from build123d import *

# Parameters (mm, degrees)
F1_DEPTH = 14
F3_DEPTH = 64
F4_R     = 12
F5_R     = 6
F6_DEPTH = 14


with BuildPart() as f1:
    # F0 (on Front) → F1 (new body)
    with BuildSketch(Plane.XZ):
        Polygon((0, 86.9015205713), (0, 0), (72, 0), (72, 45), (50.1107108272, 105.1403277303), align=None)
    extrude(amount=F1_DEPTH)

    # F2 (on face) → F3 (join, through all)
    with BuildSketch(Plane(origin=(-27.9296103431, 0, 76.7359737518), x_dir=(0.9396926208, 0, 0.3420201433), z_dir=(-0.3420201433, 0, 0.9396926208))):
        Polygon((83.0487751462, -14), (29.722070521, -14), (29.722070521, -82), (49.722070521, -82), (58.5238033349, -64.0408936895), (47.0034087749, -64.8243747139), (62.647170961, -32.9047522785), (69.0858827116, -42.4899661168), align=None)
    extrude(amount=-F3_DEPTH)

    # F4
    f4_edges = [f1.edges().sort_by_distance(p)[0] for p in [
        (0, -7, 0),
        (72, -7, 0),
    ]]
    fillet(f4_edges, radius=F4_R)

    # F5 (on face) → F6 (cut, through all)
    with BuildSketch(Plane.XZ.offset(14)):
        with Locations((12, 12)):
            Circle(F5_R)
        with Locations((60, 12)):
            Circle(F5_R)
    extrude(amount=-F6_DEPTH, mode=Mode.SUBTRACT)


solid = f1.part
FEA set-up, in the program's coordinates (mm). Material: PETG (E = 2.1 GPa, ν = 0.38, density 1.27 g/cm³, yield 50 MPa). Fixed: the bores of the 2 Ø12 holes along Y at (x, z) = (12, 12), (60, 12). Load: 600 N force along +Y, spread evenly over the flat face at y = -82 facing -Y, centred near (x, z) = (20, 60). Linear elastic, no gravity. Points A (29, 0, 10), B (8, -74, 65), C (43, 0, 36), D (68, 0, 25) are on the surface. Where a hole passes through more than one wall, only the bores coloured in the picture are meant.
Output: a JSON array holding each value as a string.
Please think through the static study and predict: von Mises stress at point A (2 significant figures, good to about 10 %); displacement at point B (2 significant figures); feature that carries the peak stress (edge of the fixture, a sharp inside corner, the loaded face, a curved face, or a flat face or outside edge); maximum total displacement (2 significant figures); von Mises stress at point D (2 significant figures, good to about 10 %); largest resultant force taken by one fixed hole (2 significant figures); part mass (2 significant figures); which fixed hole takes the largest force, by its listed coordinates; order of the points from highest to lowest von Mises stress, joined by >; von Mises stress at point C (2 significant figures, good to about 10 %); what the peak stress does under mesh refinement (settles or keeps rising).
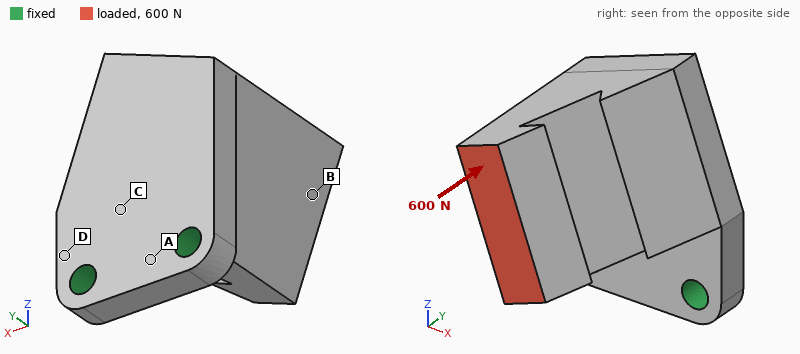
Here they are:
["2.8 MPa", "1.3 mm", "edge of the fixture", "1.6 mm", "7.6 MPa", "480 N", "290 g", "(12, 12)", "D > C > A > B", "5.1 MPa", "keeps rising"]
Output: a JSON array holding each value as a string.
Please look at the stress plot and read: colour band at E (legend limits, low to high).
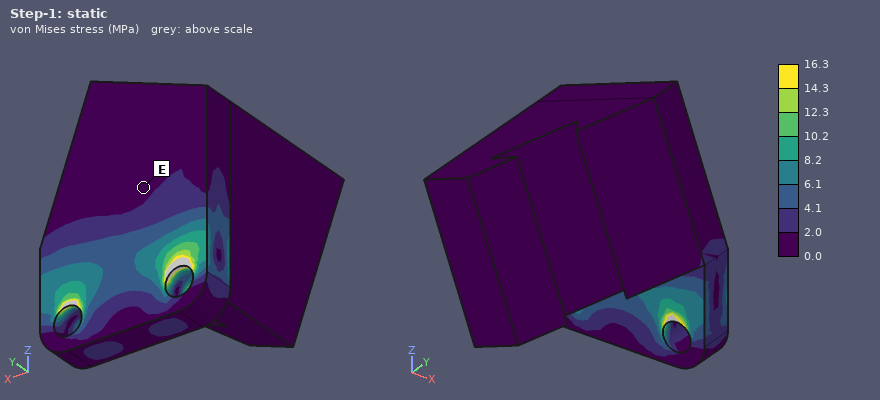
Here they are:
["0.0 to 2.0 MPa"]
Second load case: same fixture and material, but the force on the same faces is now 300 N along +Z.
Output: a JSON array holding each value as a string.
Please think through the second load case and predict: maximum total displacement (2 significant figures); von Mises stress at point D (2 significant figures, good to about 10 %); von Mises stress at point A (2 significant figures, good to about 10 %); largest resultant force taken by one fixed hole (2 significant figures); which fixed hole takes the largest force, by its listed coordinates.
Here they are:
["1.8 mm", "8.3 MPa", "2.4 MPa", "260 N", "(12, 12)"]
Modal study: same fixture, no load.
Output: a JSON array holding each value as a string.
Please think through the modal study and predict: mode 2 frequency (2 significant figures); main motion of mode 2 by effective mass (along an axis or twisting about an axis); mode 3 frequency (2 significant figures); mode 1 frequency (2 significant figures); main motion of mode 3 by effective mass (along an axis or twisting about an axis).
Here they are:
["520 Hz", "along X", "1200 Hz", "220 Hz", "along X"]
